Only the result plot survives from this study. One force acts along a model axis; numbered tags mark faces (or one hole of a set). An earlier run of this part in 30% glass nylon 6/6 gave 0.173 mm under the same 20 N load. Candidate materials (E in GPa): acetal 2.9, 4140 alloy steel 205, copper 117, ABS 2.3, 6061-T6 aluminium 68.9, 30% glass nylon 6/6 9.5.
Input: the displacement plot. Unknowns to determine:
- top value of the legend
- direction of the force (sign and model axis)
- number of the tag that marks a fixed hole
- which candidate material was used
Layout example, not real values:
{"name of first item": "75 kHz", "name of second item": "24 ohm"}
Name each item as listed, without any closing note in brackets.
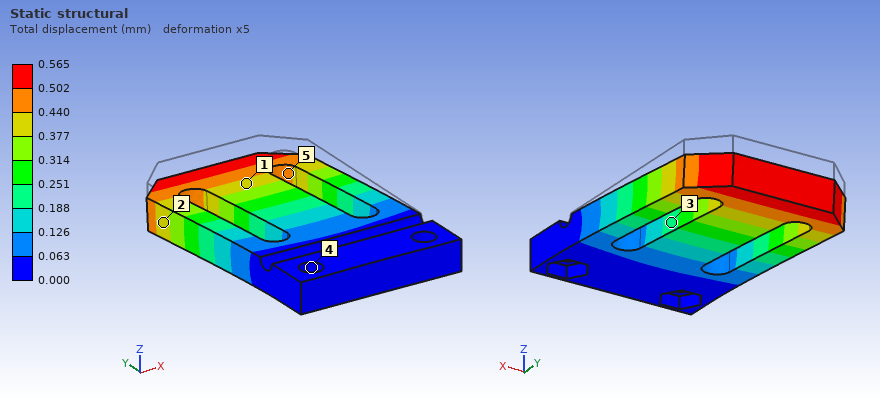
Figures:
{"top value of the legend": "0.565 mm", "direction of the force": "-Z", "number of the tag that marks a fixed hole": "4", "which candidate material was used": "acetal"}
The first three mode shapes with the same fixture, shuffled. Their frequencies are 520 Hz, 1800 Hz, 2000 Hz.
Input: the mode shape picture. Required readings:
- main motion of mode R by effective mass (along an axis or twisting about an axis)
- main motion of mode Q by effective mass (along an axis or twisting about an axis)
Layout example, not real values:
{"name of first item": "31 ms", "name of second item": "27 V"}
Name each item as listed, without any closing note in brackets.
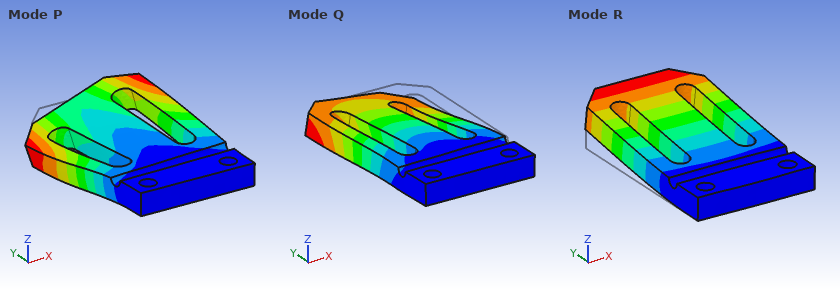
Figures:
{"main motion of mode R by effective mass": "along Z", "main motion of mode Q by effective mass": "along X"}
